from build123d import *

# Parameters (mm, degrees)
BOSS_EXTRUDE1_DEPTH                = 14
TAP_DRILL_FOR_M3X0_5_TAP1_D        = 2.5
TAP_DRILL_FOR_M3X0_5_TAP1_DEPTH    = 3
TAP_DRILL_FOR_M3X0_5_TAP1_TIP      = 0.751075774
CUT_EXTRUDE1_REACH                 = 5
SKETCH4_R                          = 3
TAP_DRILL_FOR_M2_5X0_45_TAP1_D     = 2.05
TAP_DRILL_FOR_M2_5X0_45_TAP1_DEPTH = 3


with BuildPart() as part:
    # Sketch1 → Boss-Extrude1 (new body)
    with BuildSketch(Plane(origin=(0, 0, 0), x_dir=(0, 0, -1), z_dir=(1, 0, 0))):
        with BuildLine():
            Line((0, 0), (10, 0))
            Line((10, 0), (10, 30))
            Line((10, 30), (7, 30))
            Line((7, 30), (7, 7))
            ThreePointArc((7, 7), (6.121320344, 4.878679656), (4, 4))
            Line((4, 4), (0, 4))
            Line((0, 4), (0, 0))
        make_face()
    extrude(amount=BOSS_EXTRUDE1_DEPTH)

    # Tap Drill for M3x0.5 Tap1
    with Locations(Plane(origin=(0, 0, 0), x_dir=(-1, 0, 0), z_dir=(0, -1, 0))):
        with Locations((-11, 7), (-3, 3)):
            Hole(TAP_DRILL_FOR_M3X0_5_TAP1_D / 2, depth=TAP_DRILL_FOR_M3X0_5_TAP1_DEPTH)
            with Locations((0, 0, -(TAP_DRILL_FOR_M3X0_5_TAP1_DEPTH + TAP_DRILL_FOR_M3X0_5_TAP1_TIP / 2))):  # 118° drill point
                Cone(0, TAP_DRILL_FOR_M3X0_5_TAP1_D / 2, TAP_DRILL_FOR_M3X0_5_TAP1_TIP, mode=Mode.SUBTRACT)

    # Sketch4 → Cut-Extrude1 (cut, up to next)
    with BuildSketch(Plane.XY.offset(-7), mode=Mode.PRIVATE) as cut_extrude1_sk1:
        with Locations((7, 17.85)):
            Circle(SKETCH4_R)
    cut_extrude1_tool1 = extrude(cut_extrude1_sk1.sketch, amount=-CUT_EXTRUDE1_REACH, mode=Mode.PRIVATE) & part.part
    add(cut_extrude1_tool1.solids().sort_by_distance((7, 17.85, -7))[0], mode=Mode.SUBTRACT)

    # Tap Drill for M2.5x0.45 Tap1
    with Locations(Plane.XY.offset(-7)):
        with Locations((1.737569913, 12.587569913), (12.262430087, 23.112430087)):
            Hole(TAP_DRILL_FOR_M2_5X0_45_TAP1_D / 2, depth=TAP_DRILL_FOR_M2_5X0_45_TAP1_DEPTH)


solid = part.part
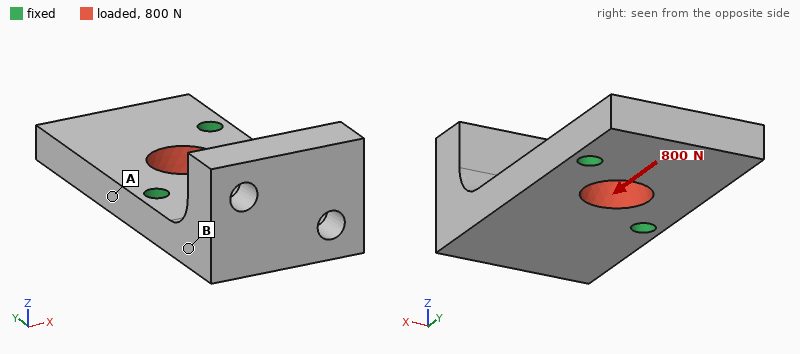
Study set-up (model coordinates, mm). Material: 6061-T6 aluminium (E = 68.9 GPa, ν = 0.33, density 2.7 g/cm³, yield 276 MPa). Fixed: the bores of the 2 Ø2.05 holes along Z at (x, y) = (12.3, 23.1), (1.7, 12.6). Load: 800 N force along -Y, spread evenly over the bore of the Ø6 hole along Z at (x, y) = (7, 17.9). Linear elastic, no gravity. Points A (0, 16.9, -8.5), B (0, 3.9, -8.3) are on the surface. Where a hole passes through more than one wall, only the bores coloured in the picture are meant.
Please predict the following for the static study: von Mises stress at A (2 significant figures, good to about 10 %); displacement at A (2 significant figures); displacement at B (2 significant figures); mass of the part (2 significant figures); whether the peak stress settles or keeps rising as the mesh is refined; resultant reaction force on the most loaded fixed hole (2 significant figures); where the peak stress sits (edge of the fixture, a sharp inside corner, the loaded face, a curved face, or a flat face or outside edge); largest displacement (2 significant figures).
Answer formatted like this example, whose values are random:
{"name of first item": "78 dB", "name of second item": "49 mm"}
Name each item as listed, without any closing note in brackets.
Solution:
{"von Mises stress at A": "19 MPa", "displacement at A": "0.99 µm", "displacement at B": "1.5 µm", "mass of the part": "4.2 g", "whether the peak stress settles or keeps rising as the mesh is refined": "keeps rising", "resultant reaction force on the most loaded fixed hole": "400 N", "where the peak stress sits": "edge of the fixture", "largest displacement": "3.7 µm"}
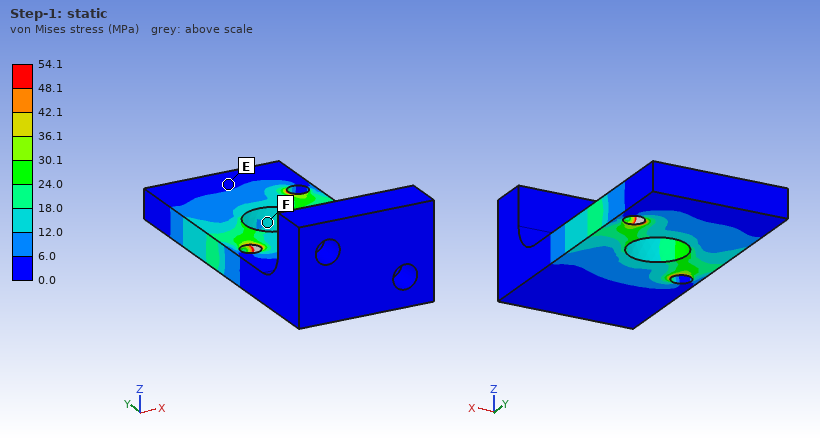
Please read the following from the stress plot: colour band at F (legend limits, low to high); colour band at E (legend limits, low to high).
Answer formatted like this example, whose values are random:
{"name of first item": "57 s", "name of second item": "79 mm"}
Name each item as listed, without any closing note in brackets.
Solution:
{"colour band at F": "12.0 to 18.0 MPa", "colour band at E": "0.0 to 6.0 MPa"}
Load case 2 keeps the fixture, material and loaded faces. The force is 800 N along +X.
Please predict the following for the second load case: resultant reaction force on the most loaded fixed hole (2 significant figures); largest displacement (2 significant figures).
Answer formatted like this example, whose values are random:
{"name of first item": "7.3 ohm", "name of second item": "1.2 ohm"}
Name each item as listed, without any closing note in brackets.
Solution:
{"resultant reaction force on the most loaded fixed hole": "400 N", "largest displacement": "3.4 µm"}
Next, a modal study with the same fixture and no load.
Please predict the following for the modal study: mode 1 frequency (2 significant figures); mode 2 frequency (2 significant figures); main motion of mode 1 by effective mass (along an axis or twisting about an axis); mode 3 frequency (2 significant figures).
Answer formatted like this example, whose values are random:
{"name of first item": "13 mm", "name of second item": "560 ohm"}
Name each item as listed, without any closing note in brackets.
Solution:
{"mode 1 frequency": "5800 Hz", "mode 2 frequency": "12 kHz", "main motion of mode 1 by effective mass": "along Z", "mode 3 frequency": "18 kHz"}
